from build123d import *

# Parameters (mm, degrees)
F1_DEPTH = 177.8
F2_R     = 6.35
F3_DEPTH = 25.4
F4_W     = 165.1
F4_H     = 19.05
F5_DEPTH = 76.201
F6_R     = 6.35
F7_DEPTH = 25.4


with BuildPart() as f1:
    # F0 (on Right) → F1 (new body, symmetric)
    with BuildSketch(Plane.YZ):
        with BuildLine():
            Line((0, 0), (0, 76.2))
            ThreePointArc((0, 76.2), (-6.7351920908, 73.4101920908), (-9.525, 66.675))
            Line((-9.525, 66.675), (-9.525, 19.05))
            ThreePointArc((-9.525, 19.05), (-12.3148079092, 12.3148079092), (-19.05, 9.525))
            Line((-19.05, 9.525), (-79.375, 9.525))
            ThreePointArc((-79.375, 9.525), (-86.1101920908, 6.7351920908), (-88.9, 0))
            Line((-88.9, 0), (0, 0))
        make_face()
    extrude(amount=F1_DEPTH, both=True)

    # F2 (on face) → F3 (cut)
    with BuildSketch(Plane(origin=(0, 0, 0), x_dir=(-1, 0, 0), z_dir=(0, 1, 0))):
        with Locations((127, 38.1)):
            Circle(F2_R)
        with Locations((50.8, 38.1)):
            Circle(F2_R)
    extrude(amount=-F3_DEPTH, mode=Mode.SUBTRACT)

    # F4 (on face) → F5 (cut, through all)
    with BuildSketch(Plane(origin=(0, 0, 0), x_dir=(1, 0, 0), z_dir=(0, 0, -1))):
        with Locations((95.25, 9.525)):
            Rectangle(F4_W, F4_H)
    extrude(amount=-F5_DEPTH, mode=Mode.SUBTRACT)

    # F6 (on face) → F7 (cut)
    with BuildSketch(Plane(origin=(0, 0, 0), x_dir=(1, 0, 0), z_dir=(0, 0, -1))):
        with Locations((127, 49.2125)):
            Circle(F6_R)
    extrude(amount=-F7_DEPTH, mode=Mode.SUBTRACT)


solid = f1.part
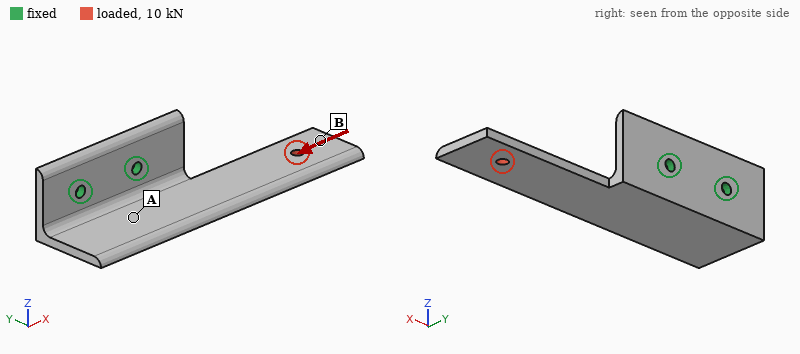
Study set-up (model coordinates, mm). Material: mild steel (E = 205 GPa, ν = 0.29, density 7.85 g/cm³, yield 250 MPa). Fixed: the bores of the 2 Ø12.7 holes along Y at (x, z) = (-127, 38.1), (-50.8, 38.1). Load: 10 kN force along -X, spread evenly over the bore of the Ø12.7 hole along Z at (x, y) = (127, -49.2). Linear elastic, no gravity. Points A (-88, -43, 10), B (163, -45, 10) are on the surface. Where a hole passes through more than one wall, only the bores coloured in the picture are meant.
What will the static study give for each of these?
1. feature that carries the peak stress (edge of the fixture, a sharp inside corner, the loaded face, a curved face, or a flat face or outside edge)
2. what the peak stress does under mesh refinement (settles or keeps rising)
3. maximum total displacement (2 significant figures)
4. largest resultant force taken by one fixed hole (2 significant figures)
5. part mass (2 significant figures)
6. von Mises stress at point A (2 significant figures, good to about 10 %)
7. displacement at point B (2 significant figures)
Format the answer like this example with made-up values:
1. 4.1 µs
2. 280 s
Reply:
1. edge of the fixture
2. keeps rising
3. 0.25 mm
4. 8.1 kN
5. 3.0 kg
6. 25 MPa
7. 0.21 mm
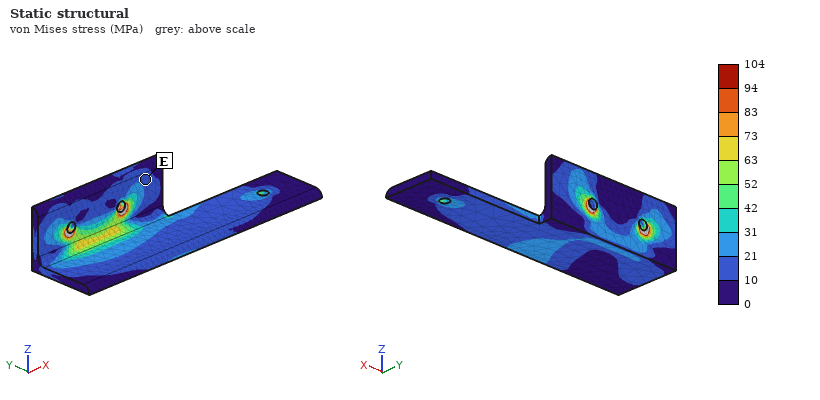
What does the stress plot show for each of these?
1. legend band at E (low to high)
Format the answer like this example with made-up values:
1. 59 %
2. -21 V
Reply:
1. 10 to 21 MPa
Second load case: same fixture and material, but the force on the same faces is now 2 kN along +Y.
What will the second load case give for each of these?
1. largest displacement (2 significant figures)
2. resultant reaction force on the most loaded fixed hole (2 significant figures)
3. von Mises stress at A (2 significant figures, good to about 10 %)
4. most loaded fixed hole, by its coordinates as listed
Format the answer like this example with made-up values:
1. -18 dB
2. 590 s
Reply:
1. 0.38 mm
2. 5.8 kN
3. 24 MPa
4. (-50.8, 38.1)
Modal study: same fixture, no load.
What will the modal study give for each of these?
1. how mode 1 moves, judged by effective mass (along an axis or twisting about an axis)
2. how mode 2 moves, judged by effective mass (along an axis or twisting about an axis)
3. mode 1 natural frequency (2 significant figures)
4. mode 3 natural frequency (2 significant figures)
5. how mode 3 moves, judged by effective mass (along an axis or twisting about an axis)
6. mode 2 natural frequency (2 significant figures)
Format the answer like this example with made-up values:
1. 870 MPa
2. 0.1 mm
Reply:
1. along Z
2. along Y
3. 190 Hz
4. 680 Hz
5. along Z
6. 510 Hz
